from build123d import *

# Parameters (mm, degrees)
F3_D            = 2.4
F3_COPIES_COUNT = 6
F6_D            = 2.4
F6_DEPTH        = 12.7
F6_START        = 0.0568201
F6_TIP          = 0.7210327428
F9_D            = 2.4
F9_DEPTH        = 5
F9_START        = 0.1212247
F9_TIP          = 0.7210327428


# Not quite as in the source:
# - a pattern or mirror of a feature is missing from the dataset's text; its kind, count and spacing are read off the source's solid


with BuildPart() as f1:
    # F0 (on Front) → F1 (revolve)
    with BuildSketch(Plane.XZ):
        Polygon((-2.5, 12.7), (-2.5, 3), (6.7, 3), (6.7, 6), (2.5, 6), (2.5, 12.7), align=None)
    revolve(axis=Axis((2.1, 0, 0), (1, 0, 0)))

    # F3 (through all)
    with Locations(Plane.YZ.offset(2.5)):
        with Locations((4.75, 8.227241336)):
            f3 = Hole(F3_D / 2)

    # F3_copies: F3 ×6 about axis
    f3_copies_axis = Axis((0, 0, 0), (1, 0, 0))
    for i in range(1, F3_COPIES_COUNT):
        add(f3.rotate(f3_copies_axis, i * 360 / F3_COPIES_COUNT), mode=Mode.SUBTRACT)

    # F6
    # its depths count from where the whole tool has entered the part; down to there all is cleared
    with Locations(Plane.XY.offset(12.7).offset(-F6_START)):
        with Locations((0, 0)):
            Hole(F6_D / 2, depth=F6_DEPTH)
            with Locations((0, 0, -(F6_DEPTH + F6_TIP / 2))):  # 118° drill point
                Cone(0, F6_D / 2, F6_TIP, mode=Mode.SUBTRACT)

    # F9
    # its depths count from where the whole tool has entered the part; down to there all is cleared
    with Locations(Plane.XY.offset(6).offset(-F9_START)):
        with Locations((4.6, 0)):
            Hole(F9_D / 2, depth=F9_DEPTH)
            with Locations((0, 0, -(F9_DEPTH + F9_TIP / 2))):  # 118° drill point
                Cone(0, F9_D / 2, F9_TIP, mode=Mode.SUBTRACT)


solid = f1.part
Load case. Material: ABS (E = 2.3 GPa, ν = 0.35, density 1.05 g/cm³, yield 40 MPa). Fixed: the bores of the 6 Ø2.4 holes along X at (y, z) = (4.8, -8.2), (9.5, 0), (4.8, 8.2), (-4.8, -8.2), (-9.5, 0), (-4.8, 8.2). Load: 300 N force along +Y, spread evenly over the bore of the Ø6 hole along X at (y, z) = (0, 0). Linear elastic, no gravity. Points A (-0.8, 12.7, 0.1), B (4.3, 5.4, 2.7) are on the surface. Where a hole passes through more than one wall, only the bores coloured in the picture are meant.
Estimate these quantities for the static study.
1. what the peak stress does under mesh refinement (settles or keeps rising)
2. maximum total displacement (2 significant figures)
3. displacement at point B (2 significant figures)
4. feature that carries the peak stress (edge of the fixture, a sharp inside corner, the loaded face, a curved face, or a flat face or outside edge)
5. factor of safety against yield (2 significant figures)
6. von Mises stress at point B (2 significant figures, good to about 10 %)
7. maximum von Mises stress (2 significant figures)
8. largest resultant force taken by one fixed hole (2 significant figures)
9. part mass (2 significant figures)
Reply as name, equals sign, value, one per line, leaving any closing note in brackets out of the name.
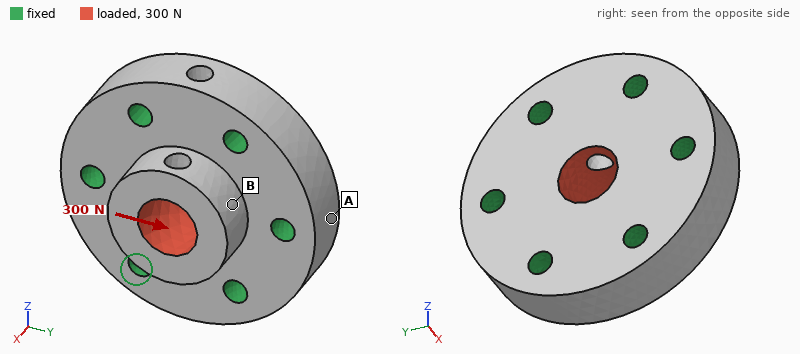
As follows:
what the peak stress does under mesh refinement = settles
maximum total displacement = 22 µm
displacement at point B = 13 µm
feature that carries the peak stress = the loaded face
factor of safety against yield = 4.5
von Mises stress at point B = 1.8 MPa
maximum von Mises stress = 8.8 MPa
largest resultant force taken by one fixed hole = 83 N
part mass = 2.7 g
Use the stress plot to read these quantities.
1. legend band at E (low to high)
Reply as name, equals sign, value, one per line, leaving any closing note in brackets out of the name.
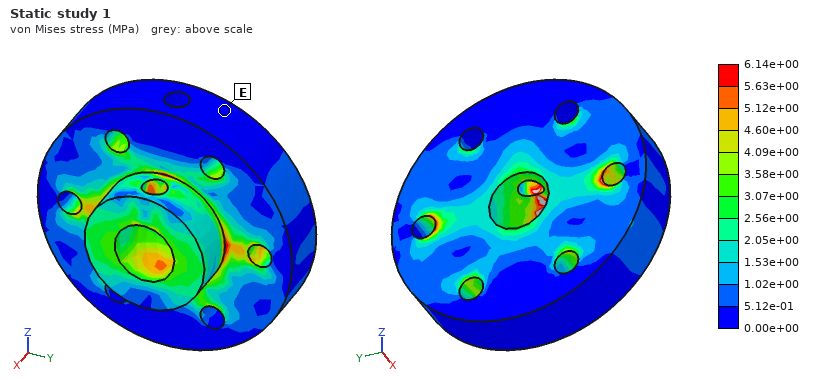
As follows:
legend band at E = 0.00e+00 to 5.12e-01 MPa
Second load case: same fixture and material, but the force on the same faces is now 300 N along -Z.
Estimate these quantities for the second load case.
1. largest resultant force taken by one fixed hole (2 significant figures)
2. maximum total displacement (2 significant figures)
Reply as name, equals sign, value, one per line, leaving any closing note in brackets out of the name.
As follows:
largest resultant force taken by one fixed hole = 73 N
maximum total displacement = 21 µm
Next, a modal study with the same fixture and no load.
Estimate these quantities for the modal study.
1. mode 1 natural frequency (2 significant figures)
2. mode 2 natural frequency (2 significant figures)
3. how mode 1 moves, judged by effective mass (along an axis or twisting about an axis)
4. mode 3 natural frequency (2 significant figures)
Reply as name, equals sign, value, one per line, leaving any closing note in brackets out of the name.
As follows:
mode 1 natural frequency = 25 kHz
mode 2 natural frequency = 26 kHz
how mode 1 moves, judged by effective mass = along X
mode 3 natural frequency = 27 kHz
